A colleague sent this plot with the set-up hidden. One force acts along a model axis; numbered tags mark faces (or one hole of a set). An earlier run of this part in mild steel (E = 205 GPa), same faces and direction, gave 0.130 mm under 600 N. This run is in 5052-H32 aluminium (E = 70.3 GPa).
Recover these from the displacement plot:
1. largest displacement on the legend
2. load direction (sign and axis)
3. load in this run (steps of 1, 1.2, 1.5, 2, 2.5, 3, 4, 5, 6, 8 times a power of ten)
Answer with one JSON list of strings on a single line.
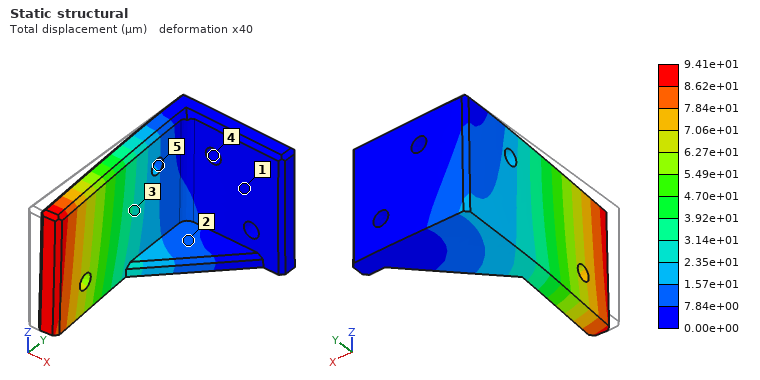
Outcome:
["9.41e+01 µm", "+X", "150 N"]
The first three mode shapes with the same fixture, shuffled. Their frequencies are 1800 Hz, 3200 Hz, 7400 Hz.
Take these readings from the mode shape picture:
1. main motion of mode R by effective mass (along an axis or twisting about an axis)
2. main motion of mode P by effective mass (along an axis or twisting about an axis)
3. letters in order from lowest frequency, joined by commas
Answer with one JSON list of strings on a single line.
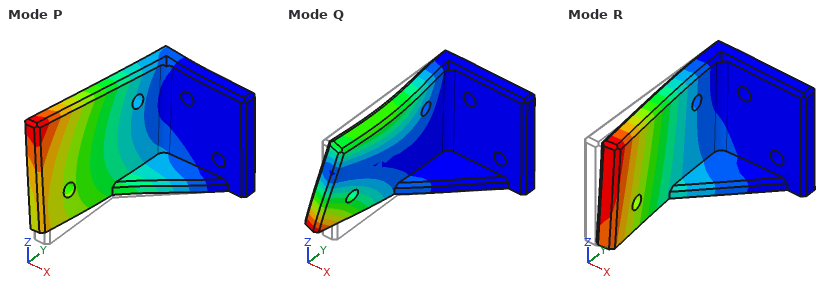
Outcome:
["along X", "along Z", "R, P, Q"]
